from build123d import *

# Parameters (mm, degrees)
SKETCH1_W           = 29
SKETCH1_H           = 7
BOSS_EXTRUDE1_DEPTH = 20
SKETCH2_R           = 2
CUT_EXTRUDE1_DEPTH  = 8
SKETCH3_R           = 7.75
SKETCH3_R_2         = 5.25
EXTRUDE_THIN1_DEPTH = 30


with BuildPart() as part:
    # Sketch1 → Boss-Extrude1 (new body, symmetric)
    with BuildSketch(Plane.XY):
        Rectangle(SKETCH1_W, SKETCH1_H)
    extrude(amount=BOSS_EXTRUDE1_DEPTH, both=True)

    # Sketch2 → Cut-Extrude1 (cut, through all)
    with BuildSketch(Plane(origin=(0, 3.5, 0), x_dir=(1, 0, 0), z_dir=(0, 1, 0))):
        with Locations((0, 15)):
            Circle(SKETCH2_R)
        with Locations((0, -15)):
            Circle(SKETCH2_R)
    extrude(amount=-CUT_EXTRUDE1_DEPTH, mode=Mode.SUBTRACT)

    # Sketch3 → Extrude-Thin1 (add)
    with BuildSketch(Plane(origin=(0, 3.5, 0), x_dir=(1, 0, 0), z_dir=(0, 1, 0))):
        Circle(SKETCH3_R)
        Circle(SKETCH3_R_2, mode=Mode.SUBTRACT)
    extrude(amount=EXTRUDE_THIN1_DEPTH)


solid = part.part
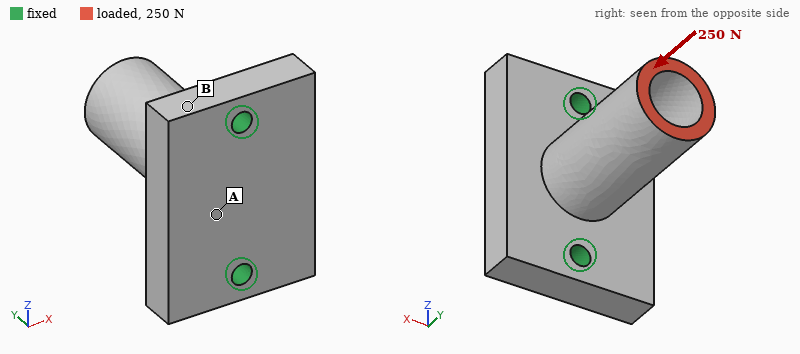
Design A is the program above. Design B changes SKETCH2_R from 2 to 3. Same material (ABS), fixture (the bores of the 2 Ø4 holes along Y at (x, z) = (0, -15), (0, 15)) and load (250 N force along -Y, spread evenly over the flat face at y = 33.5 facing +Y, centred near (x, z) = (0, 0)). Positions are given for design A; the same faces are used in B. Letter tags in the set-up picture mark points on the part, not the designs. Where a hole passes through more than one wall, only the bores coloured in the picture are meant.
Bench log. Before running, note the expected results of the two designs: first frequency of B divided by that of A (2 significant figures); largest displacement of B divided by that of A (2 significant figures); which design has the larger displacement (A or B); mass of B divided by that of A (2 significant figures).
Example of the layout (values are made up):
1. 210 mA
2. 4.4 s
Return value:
1. 1.1
2. 0.89
3. A
4. 0.98
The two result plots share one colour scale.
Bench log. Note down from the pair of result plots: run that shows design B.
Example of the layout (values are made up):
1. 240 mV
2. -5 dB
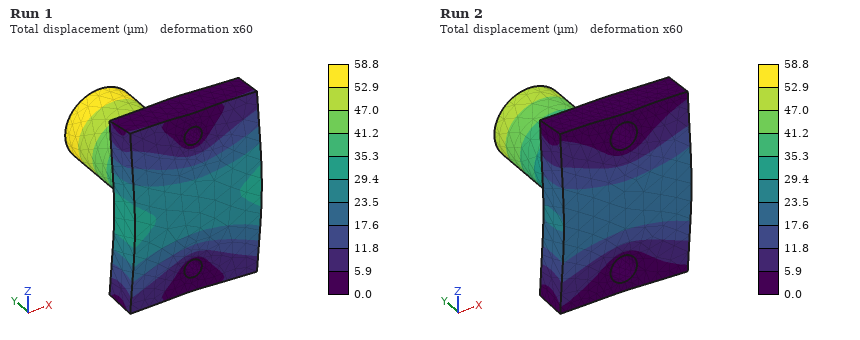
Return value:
1. Run 2
